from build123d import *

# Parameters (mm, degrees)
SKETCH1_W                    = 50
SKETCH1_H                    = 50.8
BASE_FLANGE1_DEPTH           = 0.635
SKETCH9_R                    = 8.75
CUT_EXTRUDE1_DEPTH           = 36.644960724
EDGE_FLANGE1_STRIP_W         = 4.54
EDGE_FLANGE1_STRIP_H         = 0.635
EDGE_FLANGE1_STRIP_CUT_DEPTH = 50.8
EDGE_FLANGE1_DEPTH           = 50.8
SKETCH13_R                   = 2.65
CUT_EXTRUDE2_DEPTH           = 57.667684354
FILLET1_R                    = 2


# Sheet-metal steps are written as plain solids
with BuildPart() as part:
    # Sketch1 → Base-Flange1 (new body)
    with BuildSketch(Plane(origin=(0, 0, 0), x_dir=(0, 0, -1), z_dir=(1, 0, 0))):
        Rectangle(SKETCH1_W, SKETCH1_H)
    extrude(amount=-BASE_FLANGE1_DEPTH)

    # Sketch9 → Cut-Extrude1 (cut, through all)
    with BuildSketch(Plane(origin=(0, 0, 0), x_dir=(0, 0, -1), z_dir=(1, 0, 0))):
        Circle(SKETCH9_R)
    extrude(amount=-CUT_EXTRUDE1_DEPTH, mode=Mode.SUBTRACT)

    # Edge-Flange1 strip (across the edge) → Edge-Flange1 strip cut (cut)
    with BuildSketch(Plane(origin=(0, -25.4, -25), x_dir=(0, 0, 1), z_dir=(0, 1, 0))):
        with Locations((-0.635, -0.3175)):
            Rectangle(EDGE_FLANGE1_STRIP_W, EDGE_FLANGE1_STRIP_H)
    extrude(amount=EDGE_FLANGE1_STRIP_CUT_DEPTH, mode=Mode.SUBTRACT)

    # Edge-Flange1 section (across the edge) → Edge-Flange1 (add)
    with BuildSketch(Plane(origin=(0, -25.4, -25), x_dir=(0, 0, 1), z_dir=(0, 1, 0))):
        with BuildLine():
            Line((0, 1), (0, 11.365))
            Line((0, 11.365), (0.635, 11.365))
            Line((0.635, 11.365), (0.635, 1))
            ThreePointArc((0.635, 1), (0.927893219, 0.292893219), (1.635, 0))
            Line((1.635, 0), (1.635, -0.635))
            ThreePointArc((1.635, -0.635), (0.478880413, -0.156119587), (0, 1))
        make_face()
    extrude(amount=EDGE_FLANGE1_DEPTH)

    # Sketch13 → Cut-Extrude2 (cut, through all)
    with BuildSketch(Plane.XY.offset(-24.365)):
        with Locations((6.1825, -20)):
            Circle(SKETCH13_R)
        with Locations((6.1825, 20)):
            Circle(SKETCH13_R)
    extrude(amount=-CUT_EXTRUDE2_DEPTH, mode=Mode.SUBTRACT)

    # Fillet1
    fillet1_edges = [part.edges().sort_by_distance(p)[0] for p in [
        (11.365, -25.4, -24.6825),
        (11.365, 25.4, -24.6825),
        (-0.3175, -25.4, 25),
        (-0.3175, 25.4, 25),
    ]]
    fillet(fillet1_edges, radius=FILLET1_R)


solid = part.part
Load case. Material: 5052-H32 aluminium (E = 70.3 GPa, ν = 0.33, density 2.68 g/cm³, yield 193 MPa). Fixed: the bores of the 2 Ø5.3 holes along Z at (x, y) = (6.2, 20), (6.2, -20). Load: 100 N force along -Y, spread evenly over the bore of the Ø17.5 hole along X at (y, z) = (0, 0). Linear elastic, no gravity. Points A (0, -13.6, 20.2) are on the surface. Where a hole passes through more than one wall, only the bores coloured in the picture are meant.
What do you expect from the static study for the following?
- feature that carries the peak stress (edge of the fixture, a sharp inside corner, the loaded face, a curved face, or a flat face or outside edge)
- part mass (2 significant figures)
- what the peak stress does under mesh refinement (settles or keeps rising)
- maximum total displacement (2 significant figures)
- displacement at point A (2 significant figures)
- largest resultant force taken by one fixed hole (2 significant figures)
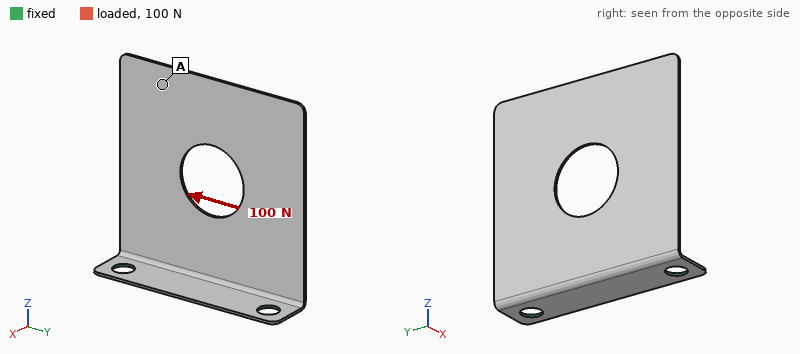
edge of the fixture
4.8 g
keeps rising
0.42 mm
0.27 mm
80 N
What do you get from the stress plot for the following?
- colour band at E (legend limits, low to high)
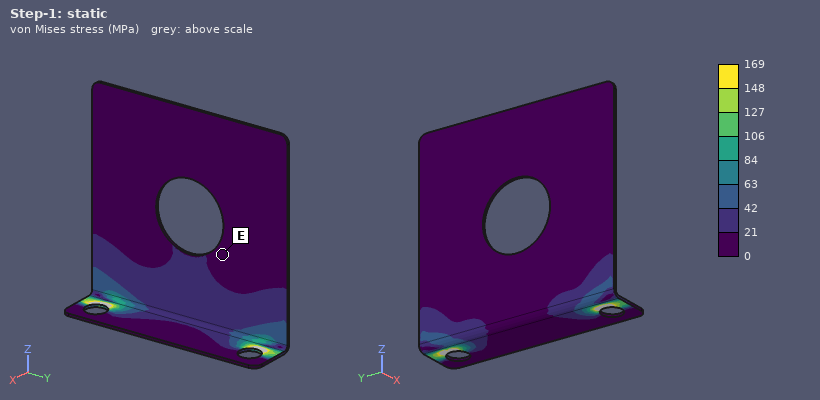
0 to 21 MPa
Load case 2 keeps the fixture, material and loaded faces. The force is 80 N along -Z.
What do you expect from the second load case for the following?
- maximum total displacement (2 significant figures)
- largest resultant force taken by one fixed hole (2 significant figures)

0.71 mm
41 N
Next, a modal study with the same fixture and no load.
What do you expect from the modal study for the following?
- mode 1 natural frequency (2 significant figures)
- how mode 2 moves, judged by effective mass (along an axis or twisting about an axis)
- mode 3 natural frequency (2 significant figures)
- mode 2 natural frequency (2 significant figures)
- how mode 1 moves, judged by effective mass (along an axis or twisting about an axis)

180 Hz
twisting about Z
1100 Hz
460 Hz
along X
